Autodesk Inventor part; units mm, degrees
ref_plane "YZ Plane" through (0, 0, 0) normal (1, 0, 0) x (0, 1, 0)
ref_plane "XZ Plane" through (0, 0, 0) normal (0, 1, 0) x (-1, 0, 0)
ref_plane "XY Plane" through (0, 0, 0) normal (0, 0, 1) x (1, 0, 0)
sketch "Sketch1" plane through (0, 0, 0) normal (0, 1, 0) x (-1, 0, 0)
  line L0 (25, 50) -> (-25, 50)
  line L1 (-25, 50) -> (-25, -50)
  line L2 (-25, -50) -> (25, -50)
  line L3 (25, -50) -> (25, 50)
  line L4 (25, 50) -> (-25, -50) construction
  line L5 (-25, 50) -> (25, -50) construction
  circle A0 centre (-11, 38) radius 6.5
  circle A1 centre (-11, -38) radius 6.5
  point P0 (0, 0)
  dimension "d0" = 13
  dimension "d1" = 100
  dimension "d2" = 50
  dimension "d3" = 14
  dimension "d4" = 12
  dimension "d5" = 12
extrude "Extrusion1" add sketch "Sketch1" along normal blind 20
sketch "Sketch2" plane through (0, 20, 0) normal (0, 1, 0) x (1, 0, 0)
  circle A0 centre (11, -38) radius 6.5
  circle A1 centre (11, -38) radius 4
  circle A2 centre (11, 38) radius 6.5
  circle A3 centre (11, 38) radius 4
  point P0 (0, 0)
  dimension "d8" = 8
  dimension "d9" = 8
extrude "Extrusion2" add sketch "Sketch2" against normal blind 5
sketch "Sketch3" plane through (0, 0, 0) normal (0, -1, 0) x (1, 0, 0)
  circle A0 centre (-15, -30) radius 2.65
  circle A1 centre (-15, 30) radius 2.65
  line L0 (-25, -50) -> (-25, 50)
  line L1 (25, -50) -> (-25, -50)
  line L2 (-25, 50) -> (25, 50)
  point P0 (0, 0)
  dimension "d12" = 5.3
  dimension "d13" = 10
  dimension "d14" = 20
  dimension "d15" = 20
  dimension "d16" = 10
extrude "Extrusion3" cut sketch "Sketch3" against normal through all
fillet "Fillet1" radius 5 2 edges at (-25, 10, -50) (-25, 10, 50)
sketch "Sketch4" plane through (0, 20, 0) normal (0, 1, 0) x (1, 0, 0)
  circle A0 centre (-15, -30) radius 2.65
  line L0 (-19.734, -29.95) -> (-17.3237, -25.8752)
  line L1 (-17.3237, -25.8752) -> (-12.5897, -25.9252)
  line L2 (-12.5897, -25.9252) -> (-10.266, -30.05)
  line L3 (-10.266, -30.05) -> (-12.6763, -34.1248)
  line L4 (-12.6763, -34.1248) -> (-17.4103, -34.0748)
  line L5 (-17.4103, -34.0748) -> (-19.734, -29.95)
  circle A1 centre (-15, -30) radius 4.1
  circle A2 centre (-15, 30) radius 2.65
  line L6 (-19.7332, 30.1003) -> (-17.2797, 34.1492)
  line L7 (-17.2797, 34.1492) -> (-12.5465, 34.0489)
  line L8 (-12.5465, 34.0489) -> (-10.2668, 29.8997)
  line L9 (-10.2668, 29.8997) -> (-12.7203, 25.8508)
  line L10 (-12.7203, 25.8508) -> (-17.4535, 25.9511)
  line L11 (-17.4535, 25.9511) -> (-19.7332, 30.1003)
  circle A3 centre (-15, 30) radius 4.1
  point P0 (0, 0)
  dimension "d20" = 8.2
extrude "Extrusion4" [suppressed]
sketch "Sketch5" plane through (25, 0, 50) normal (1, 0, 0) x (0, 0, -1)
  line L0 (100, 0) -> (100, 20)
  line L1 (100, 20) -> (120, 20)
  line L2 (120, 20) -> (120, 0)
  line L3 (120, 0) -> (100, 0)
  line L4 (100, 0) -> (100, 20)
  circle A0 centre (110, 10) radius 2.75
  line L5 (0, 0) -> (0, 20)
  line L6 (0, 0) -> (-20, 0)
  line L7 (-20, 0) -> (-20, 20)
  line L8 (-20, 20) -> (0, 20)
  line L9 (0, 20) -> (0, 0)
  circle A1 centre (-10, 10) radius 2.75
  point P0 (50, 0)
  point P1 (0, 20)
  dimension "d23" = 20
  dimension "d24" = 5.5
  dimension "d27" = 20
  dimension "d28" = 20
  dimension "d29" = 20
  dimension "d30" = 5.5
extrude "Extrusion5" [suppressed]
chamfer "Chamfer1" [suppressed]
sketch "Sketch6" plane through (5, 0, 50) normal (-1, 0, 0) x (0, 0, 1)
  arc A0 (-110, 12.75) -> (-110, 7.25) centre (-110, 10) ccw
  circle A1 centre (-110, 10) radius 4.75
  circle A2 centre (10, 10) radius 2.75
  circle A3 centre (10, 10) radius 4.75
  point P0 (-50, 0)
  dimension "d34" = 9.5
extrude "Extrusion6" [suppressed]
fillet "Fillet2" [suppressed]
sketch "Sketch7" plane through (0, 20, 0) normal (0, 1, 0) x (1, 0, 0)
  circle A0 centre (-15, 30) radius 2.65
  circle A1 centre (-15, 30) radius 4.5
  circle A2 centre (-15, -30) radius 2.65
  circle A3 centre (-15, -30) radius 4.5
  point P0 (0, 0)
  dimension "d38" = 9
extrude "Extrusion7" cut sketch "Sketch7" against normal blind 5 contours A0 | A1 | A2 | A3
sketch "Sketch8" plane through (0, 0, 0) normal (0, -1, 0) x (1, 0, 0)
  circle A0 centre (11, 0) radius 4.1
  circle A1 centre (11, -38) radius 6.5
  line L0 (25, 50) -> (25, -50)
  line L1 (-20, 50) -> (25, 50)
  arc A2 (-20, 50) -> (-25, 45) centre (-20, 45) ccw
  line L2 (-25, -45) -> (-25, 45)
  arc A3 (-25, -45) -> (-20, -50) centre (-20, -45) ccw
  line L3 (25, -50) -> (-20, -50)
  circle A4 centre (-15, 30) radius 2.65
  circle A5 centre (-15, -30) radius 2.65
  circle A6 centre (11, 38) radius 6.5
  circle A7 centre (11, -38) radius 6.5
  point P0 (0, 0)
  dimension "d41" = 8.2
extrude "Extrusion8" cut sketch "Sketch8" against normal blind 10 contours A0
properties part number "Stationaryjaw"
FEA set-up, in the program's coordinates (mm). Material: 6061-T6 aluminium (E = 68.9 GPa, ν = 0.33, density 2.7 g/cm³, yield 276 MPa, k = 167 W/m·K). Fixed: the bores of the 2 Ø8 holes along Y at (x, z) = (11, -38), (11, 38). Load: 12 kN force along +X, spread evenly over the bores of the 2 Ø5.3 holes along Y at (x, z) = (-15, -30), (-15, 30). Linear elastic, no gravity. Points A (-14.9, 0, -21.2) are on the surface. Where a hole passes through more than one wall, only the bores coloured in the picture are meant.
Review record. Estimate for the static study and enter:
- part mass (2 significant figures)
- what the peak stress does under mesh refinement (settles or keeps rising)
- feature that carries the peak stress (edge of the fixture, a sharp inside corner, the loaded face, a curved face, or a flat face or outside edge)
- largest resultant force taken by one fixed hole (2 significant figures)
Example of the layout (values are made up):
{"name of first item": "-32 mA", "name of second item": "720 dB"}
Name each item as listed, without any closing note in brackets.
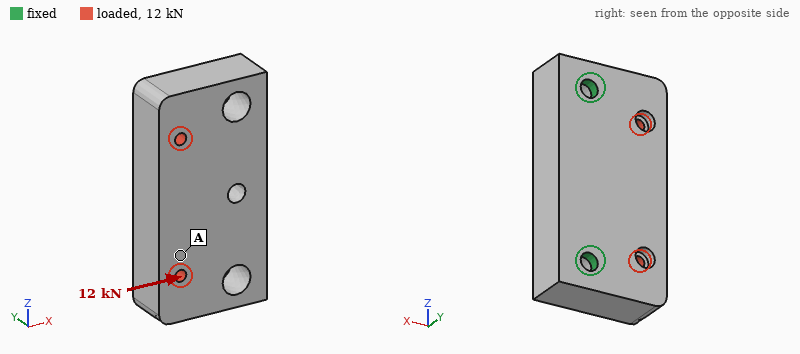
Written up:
{"part mass": "250 g", "what the peak stress does under mesh refinement": "keeps rising", "feature that carries the peak stress": "edge of the fixture", "largest resultant force taken by one fixed hole": "6.0 kN"}
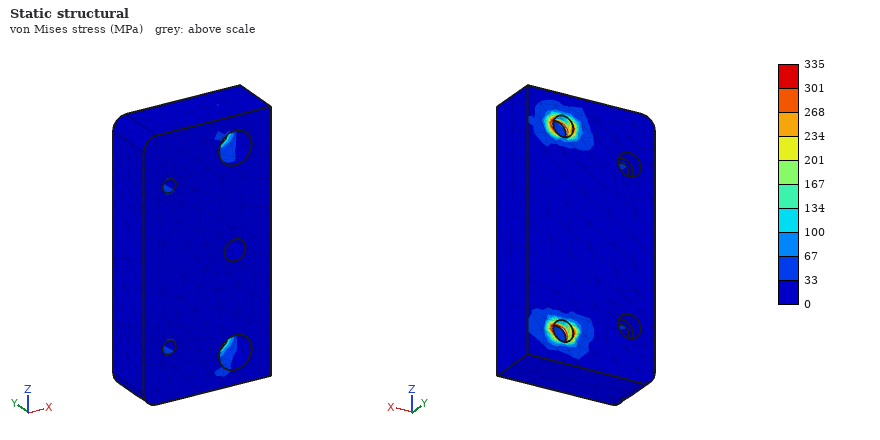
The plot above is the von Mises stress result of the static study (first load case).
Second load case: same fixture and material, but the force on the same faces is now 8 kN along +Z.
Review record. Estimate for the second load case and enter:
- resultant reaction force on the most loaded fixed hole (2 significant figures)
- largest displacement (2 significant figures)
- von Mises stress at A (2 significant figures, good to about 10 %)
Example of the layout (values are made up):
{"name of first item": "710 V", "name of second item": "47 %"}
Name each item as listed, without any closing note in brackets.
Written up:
{"resultant reaction force on the most loaded fixed hole": "4.9 kN", "largest displacement": "17 µm", "von Mises stress at A": "13 MPa"}
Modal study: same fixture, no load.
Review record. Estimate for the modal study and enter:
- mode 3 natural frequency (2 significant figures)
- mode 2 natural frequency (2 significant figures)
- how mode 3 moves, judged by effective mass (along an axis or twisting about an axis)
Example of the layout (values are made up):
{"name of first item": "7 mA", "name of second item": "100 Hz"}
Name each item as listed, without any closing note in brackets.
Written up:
{"mode 3 natural frequency": "8500 Hz", "mode 2 natural frequency": "7600 Hz", "how mode 3 moves, judged by effective mass": "along Y"}
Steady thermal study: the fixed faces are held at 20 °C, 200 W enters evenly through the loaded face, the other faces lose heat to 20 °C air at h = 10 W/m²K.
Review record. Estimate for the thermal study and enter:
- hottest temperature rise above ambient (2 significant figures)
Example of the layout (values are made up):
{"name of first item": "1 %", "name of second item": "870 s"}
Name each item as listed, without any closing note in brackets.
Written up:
{"hottest temperature rise above ambient": "46 K"}
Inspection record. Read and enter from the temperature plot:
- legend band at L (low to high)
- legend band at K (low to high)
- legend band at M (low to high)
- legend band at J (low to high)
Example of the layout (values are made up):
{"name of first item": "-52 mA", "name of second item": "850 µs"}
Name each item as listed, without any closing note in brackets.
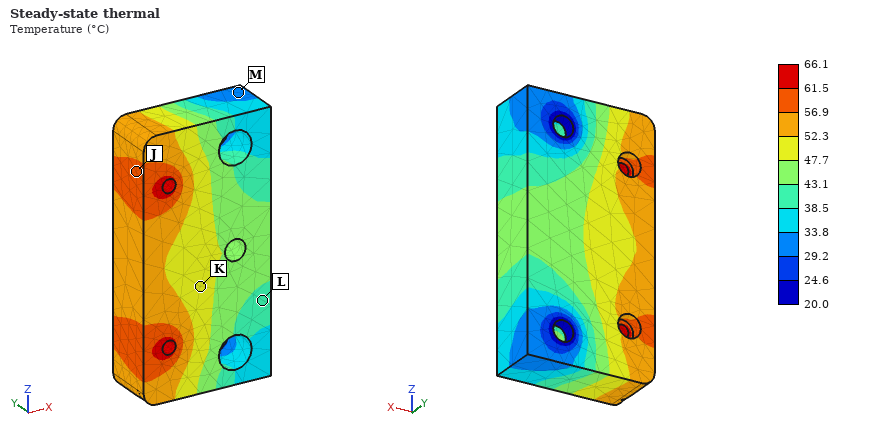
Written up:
{"legend band at L": "38.5 to 43.1 °C", "legend band at K": "47.7 to 52.3 °C", "legend band at M": "29.2 to 33.8 °C", "legend band at J": "56.9 to 61.5 °C"}
